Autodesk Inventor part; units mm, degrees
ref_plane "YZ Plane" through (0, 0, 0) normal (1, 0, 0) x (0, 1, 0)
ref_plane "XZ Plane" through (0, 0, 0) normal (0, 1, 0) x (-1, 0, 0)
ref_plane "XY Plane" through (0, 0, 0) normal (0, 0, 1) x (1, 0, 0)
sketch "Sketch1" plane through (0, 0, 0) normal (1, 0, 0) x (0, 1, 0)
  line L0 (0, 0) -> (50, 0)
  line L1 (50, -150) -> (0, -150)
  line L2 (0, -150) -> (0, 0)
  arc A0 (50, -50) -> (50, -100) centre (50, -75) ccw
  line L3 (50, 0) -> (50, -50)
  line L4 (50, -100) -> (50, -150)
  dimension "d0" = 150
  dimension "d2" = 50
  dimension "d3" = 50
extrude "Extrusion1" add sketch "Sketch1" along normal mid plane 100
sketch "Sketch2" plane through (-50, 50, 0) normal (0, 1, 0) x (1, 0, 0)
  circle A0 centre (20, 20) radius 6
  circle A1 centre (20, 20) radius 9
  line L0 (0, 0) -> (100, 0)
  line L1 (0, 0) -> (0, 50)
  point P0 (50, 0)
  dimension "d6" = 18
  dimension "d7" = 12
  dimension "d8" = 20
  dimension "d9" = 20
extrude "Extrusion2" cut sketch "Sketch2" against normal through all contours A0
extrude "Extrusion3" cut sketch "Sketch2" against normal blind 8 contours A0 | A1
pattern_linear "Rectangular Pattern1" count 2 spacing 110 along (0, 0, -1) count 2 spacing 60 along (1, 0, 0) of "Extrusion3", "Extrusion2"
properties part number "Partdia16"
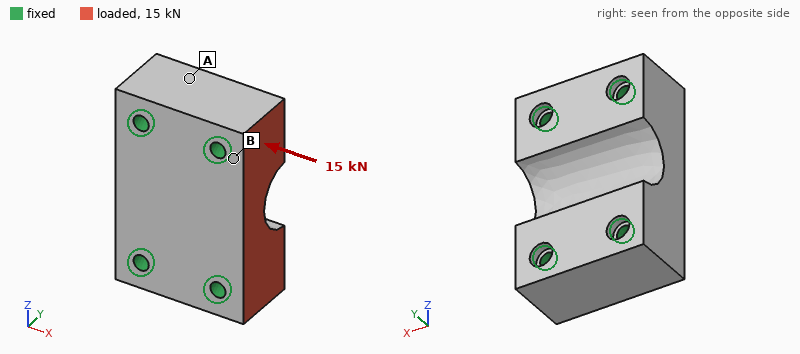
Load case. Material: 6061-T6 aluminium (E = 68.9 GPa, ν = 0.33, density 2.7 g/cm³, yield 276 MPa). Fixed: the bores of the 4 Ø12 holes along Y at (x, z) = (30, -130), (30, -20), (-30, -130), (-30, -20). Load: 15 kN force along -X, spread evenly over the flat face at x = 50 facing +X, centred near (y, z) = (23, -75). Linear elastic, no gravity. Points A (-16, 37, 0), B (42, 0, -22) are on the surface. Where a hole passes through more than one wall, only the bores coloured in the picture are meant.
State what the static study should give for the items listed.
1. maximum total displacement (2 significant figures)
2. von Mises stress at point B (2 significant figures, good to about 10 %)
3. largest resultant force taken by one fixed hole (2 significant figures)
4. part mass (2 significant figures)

2.9 µm
3.1 MPa
5.6 kN
1.7 kg
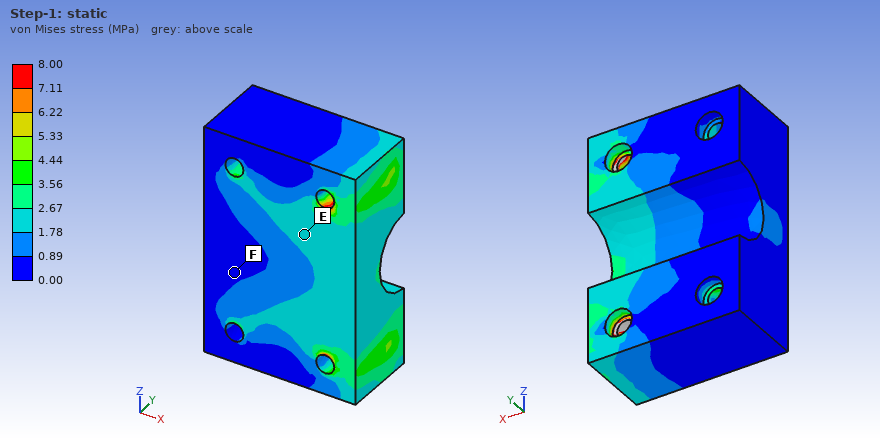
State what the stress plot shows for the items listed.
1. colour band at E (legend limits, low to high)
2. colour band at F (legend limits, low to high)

1.78 to 2.67 MPa
0.00 to 0.89 MPa
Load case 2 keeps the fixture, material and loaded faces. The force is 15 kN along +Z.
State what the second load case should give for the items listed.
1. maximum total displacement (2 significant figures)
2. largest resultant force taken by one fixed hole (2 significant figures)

4.6 µm
7.6 kN
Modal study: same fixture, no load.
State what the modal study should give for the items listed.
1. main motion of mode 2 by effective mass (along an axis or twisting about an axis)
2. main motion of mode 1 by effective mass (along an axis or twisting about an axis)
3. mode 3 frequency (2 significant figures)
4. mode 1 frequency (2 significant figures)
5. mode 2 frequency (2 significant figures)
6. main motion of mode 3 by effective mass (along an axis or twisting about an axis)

along X
along Y
15 kHz
10 kHz
12 kHz
along X
